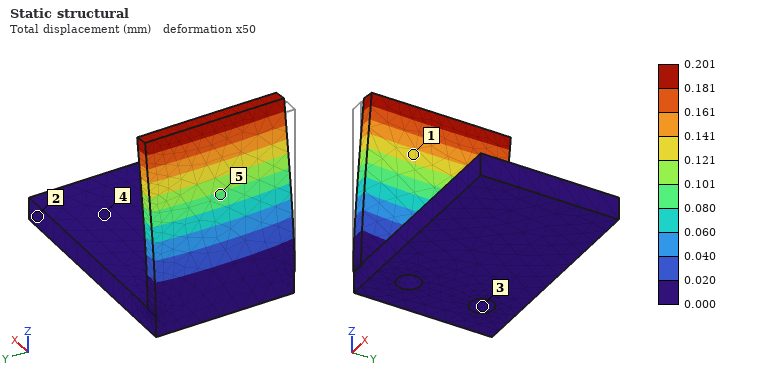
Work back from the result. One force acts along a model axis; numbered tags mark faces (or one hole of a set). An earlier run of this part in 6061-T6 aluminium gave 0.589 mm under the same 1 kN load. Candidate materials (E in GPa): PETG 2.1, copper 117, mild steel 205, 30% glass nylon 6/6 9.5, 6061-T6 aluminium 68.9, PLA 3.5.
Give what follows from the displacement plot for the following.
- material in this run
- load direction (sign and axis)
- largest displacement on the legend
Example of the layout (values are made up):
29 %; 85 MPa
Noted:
mild steel; +X; 0.201 mm
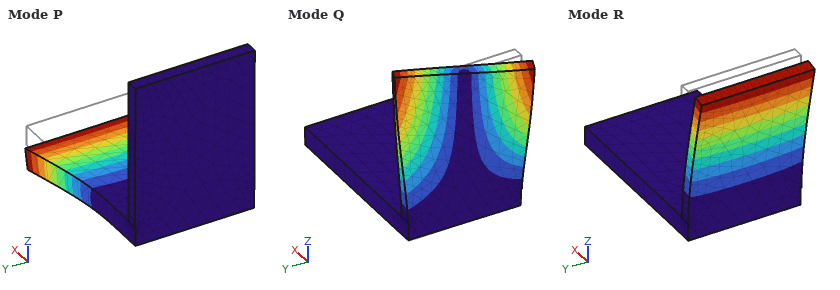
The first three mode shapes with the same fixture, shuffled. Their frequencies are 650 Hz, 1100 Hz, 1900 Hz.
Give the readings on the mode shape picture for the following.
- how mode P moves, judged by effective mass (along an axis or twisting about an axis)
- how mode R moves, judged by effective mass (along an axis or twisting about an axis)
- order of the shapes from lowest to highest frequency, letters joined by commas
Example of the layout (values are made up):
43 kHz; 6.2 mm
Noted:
along Z; along X; R, P, Q
